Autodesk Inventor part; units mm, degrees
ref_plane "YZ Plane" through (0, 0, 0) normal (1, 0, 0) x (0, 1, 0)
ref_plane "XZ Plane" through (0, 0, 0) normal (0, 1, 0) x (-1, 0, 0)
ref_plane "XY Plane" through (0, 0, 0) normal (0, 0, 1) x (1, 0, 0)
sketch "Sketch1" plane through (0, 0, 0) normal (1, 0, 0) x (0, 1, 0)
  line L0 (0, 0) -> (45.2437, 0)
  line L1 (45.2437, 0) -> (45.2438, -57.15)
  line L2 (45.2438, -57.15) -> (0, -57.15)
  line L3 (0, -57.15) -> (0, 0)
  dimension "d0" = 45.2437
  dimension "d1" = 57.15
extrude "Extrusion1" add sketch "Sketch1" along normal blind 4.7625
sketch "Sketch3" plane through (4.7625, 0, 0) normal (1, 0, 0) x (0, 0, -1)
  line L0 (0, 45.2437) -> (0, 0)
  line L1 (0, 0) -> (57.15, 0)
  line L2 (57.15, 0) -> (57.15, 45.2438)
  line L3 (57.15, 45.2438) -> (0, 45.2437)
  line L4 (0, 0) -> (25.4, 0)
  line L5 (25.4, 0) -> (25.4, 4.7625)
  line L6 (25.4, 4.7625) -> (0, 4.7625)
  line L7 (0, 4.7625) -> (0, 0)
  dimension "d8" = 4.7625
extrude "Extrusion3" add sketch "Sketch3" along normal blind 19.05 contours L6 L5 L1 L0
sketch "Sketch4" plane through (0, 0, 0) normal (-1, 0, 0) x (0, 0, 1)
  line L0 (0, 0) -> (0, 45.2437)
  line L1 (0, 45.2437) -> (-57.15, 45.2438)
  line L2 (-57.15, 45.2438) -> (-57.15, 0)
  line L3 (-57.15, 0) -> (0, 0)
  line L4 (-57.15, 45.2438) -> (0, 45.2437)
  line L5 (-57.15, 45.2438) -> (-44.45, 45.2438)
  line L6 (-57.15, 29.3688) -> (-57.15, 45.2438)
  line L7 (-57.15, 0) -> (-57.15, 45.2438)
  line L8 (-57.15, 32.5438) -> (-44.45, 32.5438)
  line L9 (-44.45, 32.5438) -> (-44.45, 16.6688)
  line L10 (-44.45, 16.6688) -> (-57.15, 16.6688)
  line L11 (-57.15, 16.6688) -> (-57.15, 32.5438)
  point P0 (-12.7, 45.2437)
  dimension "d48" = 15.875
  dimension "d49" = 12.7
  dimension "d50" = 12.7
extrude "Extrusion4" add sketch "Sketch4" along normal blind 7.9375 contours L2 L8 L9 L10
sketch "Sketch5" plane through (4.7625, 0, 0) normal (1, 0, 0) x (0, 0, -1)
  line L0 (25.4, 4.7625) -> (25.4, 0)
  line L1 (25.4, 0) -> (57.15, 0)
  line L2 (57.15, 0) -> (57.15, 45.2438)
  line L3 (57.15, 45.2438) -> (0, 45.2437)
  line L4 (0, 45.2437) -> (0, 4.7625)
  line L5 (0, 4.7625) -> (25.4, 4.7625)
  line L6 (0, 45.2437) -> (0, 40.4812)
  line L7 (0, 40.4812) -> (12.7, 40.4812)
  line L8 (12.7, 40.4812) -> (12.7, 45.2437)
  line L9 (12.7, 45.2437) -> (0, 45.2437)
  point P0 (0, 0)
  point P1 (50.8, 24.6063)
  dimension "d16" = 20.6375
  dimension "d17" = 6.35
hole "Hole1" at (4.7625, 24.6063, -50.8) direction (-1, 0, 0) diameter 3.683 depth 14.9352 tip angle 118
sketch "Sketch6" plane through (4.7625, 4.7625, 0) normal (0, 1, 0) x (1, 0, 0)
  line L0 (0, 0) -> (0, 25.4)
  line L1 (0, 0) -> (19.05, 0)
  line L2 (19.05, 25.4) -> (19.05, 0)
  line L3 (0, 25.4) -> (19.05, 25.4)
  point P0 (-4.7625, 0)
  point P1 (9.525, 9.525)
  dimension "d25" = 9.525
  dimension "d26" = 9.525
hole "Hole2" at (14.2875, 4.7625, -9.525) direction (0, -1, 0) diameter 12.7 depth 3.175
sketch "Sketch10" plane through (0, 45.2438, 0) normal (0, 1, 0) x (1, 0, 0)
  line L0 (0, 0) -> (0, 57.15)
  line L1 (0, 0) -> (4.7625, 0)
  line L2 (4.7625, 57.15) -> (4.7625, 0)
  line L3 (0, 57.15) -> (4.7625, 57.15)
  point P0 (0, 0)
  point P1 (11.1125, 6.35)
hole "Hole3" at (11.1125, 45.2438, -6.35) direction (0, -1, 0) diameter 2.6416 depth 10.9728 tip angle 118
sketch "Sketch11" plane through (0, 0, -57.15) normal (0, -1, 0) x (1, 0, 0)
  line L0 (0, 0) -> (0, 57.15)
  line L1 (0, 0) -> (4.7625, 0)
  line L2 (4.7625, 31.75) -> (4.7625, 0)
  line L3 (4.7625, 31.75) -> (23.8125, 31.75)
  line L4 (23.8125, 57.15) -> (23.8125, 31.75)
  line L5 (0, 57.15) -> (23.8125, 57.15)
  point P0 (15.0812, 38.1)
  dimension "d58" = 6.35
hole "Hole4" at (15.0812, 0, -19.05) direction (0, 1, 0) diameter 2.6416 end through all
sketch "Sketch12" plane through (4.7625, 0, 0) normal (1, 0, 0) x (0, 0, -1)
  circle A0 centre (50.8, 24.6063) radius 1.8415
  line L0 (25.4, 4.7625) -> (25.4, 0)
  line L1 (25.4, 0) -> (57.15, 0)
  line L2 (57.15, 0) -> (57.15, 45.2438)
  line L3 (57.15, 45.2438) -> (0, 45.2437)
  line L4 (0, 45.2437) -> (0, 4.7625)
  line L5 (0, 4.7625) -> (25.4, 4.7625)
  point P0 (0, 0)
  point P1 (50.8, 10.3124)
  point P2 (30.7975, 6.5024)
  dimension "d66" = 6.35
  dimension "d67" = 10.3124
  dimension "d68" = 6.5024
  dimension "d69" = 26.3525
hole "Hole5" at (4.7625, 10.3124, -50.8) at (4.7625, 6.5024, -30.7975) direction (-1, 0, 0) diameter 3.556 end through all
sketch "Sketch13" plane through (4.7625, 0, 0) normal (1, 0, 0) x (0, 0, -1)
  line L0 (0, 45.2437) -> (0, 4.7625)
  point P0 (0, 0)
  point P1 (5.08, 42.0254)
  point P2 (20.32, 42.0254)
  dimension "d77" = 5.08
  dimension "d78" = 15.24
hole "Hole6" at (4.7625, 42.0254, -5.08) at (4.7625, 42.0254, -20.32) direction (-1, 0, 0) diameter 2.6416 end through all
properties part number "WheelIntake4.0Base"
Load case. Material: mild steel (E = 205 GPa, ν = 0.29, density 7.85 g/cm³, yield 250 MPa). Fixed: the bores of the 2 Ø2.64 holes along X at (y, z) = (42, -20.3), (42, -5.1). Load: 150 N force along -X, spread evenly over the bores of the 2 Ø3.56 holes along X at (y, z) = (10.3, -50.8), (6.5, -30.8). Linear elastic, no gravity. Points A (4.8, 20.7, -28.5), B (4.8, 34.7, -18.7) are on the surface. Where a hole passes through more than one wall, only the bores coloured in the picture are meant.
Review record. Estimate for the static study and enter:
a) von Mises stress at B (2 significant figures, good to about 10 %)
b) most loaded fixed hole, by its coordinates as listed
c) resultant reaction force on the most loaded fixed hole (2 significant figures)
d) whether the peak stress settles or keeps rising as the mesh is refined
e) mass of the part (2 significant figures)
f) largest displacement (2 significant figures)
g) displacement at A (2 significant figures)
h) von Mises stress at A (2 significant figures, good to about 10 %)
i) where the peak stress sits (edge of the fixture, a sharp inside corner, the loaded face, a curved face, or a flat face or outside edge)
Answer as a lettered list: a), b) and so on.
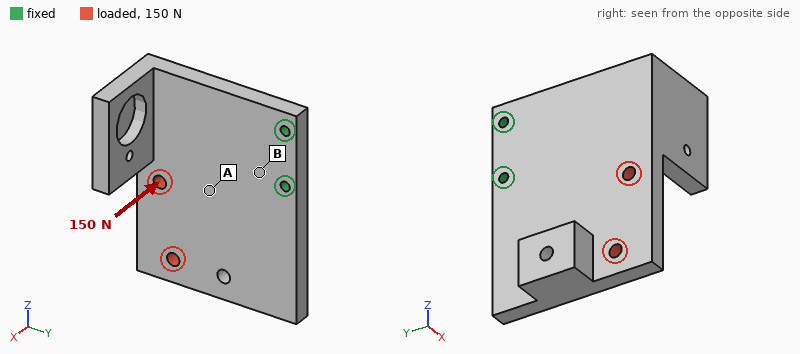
a) 39 MPa
b) (42, -20.3)
c) 270 N
d) keeps rising
e) 120 g
f) 85 µm
g) 27 µm
h) 12 MPa
i) edge of the fixture
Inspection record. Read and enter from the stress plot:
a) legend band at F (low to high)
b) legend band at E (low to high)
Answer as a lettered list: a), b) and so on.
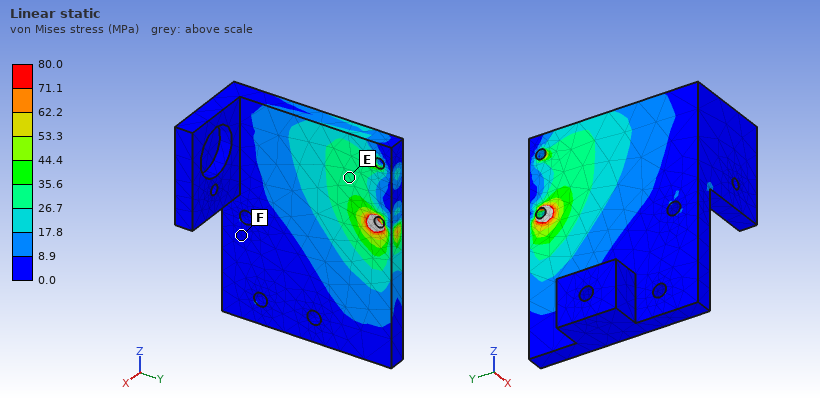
a) 0.0 to 8.9 MPa
b) 26.7 to 35.6 MPa
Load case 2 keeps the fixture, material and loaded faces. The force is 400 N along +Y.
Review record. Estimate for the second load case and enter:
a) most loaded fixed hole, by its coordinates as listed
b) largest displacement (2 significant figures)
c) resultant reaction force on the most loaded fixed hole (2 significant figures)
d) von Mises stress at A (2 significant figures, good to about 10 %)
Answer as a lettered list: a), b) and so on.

a) (42, -20.3)
b) 8.4 µm
c) 860 N
d) 5.0 MPa
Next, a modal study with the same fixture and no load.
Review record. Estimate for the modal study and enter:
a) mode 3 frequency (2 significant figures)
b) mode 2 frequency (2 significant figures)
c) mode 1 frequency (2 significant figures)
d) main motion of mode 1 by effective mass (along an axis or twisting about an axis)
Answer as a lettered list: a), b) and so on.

a) 3600 Hz
b) 1800 Hz
c) 1100 Hz
d) along X
